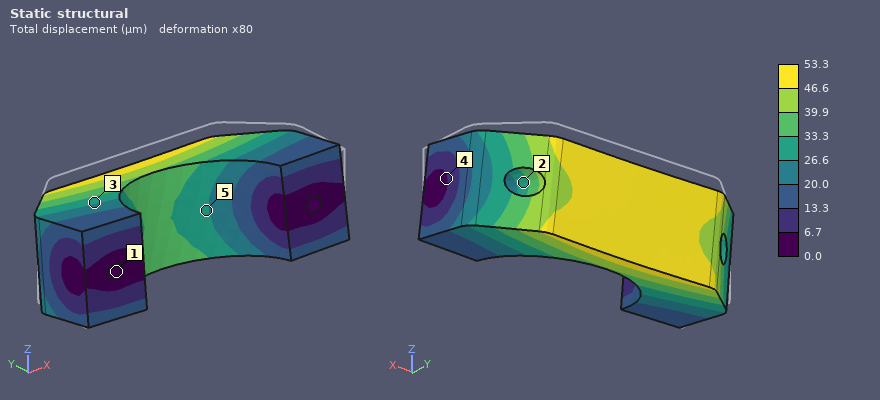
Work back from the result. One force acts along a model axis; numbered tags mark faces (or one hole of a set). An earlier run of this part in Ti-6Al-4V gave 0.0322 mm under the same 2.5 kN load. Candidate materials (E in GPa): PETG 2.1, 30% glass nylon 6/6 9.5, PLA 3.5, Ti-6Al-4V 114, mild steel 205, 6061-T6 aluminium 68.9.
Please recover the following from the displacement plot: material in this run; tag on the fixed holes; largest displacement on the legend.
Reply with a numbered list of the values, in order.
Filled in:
1. 6061-T6 aluminium
2. 1
3. 53.3 µm
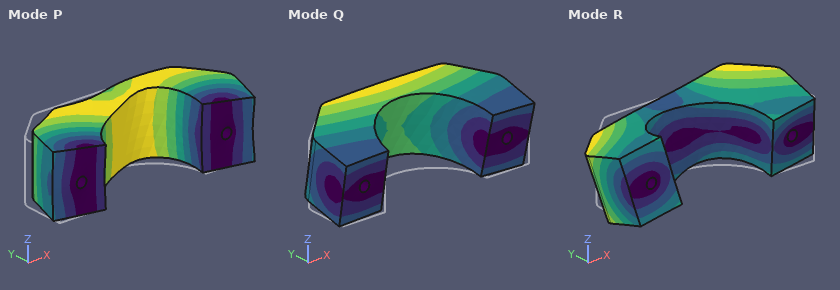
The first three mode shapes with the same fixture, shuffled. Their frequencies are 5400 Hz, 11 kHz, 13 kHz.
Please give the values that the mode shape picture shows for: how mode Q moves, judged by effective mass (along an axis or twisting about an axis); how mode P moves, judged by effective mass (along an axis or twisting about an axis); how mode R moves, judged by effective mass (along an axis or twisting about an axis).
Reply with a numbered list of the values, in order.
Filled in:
1. along Z
2. along X
3. twisting about Y
